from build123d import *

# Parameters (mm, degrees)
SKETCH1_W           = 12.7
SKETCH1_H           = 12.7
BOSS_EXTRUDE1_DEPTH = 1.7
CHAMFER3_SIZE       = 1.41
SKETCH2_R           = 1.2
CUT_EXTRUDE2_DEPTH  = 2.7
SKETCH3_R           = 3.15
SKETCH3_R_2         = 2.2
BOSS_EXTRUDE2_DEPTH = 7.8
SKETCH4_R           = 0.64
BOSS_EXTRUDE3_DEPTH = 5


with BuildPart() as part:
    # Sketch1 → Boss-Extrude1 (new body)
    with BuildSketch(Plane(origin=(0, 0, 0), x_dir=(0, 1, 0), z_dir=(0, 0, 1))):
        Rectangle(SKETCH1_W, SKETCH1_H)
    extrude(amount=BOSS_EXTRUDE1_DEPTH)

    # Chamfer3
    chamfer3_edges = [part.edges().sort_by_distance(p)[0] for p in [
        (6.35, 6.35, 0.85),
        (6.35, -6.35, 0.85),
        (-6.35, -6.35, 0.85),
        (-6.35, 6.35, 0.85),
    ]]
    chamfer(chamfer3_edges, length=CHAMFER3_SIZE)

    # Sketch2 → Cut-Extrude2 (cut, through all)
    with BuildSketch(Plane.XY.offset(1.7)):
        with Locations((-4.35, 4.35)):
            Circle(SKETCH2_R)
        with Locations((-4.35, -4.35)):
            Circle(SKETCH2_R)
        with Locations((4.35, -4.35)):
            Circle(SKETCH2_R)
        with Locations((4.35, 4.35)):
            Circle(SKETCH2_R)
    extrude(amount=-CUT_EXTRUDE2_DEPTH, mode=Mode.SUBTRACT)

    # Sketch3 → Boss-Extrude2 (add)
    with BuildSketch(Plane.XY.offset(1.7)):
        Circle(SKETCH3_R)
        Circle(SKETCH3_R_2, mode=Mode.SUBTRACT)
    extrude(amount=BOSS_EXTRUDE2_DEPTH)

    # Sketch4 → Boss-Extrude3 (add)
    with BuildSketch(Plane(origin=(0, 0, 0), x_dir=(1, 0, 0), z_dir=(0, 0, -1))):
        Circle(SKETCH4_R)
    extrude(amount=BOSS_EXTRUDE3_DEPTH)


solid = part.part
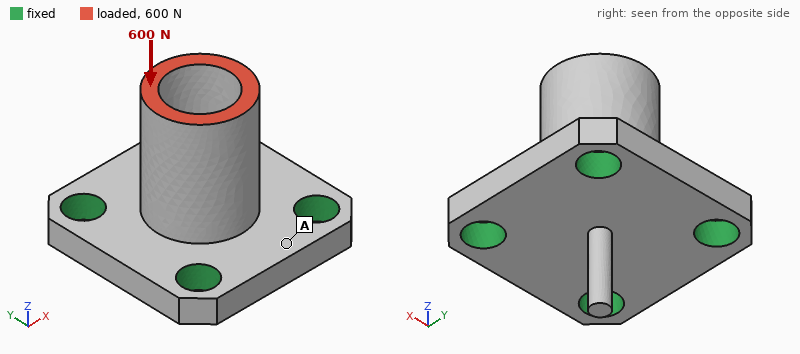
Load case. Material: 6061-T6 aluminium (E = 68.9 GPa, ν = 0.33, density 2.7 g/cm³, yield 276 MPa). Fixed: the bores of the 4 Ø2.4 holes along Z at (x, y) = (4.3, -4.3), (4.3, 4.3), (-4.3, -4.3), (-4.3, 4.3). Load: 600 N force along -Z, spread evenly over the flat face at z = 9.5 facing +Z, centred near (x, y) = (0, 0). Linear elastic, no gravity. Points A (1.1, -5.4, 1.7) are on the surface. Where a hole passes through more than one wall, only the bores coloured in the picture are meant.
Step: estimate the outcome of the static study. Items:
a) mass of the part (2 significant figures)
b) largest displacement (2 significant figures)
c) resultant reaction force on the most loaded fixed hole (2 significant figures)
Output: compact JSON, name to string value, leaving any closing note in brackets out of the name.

{"mass of the part": "0.99 g", "largest displacement": "8.8 µm", "resultant reaction force on the most loaded fixed hole": "150 N"}
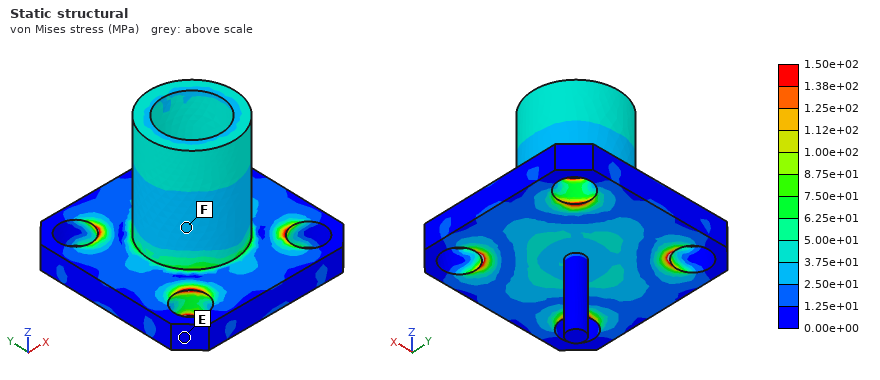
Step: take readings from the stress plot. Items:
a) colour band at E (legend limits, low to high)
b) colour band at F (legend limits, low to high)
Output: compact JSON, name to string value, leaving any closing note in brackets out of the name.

{"colour band at E": "0.00e+00 to 1.25e+01 MPa", "colour band at F": "2.50e+01 to 3.75e+01 MPa"}
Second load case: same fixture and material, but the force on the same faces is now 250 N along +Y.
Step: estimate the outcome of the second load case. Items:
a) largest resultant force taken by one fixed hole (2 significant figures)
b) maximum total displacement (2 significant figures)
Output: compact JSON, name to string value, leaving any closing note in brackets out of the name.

{"largest resultant force taken by one fixed hole": "170 N", "maximum total displacement": "37 µm"}
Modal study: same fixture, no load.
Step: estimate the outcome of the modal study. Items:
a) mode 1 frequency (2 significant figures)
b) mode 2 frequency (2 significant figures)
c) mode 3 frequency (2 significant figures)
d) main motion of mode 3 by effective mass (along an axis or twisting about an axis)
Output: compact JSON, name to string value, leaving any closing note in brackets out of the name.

{"mode 1 frequency": "31 kHz", "mode 2 frequency": "31 kHz", "mode 3 frequency": "40 kHz", "main motion of mode 3 by effective mass": "along X"}
